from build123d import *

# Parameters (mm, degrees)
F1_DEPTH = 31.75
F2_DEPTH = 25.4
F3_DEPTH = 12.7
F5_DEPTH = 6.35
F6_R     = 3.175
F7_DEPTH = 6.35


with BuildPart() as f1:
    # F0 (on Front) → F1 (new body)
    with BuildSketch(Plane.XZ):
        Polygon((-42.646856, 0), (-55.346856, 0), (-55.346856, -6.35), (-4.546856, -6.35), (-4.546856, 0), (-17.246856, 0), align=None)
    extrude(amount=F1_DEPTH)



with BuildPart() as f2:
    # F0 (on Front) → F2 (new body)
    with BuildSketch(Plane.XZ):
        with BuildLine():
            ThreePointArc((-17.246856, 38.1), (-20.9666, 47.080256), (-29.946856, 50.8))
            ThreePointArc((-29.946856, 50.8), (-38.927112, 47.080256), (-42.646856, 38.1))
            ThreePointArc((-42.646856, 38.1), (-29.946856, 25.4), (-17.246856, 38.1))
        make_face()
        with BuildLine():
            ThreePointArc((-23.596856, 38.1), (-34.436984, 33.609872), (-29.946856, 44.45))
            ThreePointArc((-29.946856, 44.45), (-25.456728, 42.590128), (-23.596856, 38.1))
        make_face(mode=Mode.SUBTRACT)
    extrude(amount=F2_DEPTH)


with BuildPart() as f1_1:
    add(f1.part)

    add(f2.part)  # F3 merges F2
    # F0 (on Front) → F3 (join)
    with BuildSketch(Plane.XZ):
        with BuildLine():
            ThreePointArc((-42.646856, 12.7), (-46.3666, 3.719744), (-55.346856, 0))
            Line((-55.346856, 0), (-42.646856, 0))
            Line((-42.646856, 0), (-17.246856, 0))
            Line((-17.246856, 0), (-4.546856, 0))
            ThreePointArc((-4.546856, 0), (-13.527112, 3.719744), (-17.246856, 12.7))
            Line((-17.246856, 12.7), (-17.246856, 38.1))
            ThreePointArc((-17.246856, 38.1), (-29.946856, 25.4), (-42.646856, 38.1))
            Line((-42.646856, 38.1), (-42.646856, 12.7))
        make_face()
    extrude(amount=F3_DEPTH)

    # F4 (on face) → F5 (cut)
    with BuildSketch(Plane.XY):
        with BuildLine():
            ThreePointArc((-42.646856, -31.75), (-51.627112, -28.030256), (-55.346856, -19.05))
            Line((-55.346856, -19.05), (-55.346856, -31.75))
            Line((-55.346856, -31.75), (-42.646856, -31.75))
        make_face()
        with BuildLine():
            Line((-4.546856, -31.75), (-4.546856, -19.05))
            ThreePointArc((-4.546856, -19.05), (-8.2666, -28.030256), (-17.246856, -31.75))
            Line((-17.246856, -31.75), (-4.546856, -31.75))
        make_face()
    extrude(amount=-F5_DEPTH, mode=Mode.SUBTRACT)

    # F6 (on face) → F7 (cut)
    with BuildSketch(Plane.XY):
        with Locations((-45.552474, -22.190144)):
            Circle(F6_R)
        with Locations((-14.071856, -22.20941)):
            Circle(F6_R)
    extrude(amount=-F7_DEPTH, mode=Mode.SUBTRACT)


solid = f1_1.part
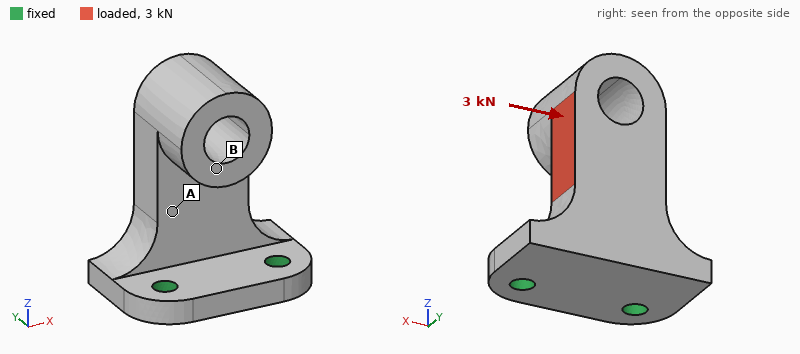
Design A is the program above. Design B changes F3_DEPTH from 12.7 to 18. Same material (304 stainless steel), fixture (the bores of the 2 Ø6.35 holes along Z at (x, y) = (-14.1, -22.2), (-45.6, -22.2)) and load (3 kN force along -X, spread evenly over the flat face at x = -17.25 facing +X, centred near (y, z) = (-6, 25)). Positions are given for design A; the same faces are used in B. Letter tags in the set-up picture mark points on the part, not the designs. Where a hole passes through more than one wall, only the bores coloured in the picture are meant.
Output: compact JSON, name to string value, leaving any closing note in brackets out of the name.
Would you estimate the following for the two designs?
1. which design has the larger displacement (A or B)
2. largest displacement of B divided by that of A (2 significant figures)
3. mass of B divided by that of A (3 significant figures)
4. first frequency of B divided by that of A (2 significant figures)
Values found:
{"which design has the larger displacement": "A", "largest displacement of B divided by that of A": "0.47", "mass of B divided by that of A": "1.14", "first frequency of B divided by that of A": "1.3"}
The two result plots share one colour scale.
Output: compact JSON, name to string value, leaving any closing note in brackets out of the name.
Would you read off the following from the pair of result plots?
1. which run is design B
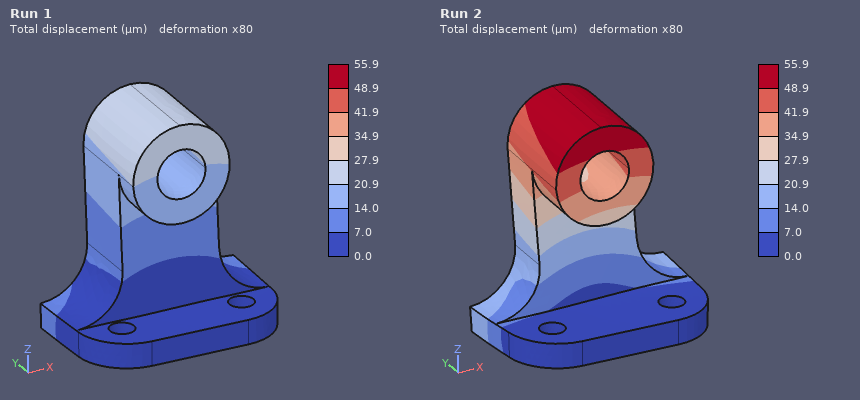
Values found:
{"which run is design B": "Run 1"}
